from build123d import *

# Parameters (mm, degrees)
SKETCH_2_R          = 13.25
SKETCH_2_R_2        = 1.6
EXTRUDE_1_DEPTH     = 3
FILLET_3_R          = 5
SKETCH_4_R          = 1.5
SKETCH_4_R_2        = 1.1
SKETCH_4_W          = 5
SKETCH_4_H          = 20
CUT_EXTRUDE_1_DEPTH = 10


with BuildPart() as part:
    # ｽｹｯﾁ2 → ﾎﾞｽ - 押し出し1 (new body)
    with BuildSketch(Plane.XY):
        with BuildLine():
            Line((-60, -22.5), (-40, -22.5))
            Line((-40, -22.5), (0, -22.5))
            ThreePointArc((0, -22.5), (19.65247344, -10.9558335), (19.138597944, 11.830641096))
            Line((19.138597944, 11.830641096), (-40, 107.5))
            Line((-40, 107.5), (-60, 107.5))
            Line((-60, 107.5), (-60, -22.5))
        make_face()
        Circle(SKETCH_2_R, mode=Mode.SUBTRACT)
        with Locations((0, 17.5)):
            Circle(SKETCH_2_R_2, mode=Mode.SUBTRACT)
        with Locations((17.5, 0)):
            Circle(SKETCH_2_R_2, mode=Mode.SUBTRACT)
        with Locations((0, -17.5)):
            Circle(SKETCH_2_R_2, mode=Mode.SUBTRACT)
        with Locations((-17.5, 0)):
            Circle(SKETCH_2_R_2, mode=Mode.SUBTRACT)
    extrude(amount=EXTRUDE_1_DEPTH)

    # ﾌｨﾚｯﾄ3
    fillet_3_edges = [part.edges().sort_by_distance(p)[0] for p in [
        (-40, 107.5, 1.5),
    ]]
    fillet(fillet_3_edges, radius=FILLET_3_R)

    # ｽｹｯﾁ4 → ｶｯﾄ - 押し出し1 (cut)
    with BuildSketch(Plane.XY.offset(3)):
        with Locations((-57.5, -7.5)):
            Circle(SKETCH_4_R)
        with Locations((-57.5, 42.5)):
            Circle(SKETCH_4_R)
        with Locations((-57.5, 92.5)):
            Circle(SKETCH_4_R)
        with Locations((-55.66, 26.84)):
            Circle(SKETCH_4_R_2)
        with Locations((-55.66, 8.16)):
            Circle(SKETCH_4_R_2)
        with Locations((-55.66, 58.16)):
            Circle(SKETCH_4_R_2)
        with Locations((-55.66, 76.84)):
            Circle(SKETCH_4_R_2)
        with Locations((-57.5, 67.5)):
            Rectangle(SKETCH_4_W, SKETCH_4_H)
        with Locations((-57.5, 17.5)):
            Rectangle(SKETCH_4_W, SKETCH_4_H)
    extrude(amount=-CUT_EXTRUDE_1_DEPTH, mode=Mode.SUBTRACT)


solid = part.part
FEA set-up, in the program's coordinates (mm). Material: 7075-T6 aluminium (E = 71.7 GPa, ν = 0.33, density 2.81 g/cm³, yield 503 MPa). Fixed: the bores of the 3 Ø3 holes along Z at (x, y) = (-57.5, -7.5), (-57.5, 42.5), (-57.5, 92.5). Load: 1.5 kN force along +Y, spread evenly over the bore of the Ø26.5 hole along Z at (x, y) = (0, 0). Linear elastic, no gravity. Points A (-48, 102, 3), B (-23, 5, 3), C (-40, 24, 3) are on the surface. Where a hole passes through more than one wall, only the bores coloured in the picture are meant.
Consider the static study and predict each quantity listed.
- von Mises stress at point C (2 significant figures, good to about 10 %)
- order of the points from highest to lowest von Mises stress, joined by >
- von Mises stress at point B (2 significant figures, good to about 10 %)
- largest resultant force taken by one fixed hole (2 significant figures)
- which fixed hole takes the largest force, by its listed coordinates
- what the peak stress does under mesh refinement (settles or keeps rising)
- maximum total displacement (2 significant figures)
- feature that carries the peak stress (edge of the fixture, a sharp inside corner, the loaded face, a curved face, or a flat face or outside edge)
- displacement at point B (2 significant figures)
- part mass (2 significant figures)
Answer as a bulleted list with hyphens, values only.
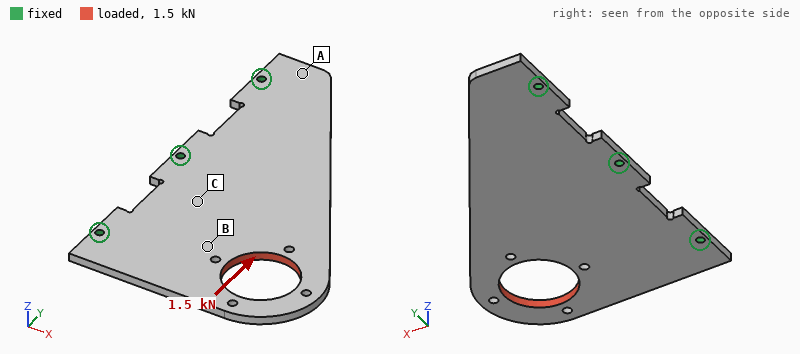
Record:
- 9.8 MPa
- B > C > A
- 18 MPa
- 1.1 kN
- (-57.5, -7.5)
- keeps rising
- 49 µm
- edge of the fixture
- 15 µm
- 56 g
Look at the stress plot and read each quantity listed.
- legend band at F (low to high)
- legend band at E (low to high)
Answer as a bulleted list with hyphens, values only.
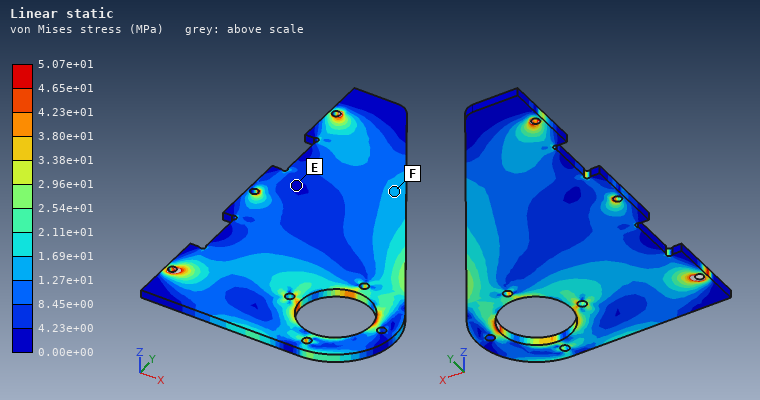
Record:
- 1.27e+01 to 1.69e+01 MPa
- 0.00e+00 to 4.23e+00 MPa
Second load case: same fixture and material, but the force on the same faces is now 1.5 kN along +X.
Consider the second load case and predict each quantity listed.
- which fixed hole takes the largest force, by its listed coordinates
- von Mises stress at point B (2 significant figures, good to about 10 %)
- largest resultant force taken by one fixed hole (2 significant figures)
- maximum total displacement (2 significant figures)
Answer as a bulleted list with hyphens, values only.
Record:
- (-57.5, -7.5)
- 10 MPa
- 1.2 kN
- 28 µm
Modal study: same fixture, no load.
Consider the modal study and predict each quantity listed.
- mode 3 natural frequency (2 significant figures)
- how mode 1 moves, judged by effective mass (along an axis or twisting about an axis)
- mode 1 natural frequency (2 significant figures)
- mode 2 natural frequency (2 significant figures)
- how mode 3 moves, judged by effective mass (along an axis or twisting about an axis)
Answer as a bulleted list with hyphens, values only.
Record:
- 2200 Hz
- along Z
- 500 Hz
- 1200 Hz
- along Z
